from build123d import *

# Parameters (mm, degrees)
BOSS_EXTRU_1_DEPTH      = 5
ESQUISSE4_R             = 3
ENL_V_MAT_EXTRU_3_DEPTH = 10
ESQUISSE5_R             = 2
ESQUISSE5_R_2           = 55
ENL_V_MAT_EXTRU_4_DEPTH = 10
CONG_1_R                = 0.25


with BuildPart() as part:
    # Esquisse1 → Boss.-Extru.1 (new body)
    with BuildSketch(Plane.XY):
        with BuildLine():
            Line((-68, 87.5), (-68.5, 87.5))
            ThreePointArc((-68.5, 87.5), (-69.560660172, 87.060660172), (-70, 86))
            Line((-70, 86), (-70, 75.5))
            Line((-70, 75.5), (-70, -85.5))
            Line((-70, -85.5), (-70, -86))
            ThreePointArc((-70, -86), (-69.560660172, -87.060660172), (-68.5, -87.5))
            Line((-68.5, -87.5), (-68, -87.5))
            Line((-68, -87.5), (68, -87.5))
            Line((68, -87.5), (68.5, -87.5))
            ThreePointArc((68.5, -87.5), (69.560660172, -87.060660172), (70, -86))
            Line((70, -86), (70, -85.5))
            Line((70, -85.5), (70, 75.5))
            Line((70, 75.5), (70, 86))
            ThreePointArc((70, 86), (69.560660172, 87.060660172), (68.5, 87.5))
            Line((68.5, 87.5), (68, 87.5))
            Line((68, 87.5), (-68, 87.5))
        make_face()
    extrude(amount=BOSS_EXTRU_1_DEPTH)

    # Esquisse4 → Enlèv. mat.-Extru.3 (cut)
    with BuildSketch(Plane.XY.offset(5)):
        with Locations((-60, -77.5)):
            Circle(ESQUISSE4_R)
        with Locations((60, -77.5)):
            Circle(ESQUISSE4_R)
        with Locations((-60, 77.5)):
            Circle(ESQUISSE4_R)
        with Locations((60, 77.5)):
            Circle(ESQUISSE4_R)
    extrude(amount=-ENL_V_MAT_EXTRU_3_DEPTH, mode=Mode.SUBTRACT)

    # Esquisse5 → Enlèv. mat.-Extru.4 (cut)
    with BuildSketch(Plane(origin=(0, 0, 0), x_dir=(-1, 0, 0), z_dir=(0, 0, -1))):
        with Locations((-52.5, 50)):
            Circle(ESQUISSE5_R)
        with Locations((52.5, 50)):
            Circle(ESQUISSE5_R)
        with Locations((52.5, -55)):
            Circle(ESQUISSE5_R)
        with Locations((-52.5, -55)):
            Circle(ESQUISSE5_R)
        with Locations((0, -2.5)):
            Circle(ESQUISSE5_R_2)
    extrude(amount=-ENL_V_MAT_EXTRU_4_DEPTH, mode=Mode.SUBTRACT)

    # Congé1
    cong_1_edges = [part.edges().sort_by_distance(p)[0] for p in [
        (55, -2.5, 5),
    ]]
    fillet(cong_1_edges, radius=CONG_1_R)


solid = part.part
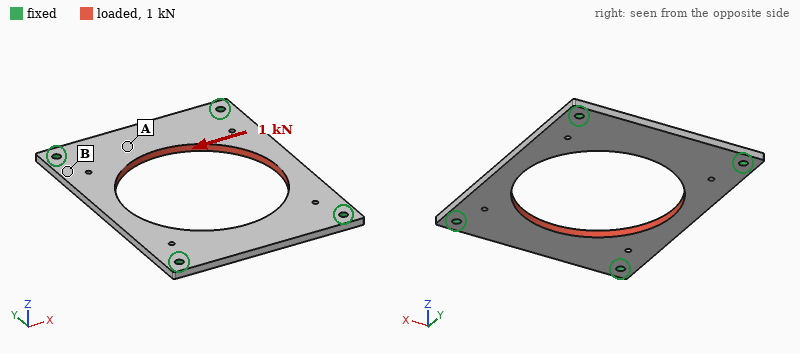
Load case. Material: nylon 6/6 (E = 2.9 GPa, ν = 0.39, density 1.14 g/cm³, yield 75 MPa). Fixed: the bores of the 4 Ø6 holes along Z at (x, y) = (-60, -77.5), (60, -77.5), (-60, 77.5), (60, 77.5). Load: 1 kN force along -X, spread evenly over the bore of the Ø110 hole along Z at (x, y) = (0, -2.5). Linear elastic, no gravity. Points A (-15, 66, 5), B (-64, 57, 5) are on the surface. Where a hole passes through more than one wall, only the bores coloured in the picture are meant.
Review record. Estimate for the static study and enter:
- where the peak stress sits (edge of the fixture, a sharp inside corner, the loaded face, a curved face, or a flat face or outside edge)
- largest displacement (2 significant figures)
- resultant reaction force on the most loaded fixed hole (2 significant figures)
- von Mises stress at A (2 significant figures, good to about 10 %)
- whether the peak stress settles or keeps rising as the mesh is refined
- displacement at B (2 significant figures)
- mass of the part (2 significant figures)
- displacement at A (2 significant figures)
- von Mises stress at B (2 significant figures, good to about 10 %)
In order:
edge of the fixture
0.16 mm
260 N
2.0 MPa
keeps rising
0.036 mm
85 g
0.034 mm
0.78 MPa
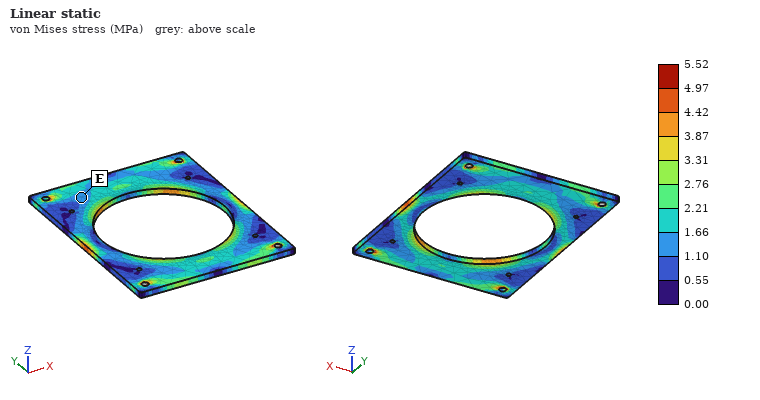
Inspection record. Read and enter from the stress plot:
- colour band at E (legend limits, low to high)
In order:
1.10 to 1.66 MPa
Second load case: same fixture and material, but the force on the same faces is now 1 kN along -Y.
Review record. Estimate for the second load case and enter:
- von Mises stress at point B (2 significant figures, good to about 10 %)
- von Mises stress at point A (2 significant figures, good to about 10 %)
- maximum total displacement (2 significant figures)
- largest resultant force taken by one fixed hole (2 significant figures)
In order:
1.7 MPa
0.85 MPa
95 µm
270 N
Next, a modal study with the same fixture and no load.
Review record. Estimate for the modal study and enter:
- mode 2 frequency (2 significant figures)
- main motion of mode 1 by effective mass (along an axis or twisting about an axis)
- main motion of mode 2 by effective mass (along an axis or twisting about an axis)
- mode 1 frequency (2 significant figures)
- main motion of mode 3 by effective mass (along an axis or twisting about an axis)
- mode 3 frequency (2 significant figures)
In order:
420 Hz
along Z
twisting about Y
380 Hz
along Z
530 Hz
